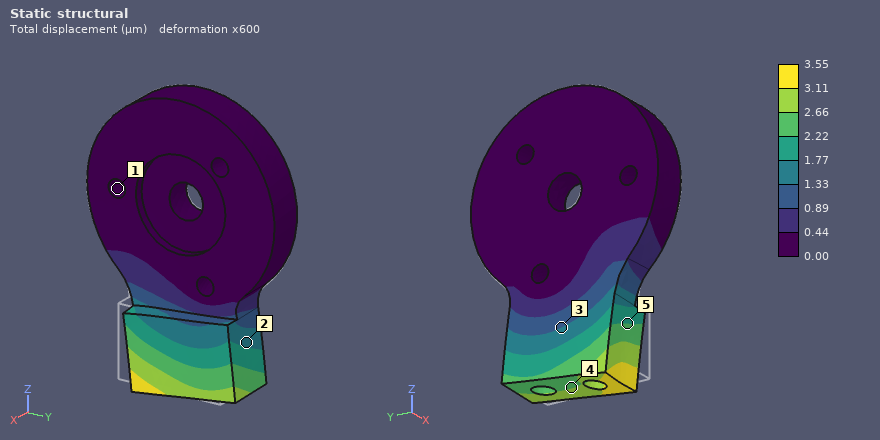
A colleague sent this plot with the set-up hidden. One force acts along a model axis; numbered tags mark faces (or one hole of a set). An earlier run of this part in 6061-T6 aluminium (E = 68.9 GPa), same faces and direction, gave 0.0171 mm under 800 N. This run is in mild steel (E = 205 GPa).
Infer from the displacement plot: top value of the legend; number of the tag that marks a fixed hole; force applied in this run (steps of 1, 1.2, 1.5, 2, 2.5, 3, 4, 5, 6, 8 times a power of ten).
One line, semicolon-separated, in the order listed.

3.55 µm; 1; 500 N
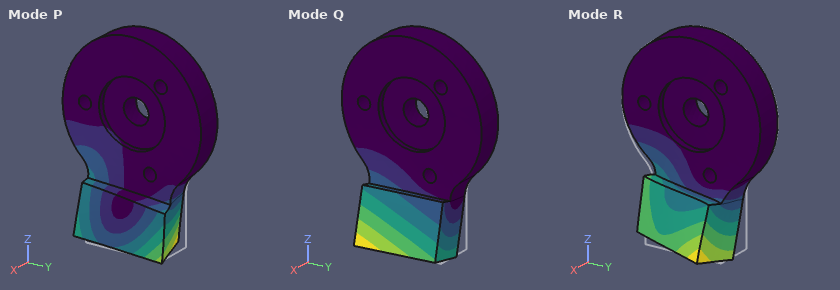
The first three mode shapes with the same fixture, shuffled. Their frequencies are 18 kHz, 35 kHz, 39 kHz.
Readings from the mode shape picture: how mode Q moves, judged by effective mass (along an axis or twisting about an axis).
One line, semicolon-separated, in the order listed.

along X
